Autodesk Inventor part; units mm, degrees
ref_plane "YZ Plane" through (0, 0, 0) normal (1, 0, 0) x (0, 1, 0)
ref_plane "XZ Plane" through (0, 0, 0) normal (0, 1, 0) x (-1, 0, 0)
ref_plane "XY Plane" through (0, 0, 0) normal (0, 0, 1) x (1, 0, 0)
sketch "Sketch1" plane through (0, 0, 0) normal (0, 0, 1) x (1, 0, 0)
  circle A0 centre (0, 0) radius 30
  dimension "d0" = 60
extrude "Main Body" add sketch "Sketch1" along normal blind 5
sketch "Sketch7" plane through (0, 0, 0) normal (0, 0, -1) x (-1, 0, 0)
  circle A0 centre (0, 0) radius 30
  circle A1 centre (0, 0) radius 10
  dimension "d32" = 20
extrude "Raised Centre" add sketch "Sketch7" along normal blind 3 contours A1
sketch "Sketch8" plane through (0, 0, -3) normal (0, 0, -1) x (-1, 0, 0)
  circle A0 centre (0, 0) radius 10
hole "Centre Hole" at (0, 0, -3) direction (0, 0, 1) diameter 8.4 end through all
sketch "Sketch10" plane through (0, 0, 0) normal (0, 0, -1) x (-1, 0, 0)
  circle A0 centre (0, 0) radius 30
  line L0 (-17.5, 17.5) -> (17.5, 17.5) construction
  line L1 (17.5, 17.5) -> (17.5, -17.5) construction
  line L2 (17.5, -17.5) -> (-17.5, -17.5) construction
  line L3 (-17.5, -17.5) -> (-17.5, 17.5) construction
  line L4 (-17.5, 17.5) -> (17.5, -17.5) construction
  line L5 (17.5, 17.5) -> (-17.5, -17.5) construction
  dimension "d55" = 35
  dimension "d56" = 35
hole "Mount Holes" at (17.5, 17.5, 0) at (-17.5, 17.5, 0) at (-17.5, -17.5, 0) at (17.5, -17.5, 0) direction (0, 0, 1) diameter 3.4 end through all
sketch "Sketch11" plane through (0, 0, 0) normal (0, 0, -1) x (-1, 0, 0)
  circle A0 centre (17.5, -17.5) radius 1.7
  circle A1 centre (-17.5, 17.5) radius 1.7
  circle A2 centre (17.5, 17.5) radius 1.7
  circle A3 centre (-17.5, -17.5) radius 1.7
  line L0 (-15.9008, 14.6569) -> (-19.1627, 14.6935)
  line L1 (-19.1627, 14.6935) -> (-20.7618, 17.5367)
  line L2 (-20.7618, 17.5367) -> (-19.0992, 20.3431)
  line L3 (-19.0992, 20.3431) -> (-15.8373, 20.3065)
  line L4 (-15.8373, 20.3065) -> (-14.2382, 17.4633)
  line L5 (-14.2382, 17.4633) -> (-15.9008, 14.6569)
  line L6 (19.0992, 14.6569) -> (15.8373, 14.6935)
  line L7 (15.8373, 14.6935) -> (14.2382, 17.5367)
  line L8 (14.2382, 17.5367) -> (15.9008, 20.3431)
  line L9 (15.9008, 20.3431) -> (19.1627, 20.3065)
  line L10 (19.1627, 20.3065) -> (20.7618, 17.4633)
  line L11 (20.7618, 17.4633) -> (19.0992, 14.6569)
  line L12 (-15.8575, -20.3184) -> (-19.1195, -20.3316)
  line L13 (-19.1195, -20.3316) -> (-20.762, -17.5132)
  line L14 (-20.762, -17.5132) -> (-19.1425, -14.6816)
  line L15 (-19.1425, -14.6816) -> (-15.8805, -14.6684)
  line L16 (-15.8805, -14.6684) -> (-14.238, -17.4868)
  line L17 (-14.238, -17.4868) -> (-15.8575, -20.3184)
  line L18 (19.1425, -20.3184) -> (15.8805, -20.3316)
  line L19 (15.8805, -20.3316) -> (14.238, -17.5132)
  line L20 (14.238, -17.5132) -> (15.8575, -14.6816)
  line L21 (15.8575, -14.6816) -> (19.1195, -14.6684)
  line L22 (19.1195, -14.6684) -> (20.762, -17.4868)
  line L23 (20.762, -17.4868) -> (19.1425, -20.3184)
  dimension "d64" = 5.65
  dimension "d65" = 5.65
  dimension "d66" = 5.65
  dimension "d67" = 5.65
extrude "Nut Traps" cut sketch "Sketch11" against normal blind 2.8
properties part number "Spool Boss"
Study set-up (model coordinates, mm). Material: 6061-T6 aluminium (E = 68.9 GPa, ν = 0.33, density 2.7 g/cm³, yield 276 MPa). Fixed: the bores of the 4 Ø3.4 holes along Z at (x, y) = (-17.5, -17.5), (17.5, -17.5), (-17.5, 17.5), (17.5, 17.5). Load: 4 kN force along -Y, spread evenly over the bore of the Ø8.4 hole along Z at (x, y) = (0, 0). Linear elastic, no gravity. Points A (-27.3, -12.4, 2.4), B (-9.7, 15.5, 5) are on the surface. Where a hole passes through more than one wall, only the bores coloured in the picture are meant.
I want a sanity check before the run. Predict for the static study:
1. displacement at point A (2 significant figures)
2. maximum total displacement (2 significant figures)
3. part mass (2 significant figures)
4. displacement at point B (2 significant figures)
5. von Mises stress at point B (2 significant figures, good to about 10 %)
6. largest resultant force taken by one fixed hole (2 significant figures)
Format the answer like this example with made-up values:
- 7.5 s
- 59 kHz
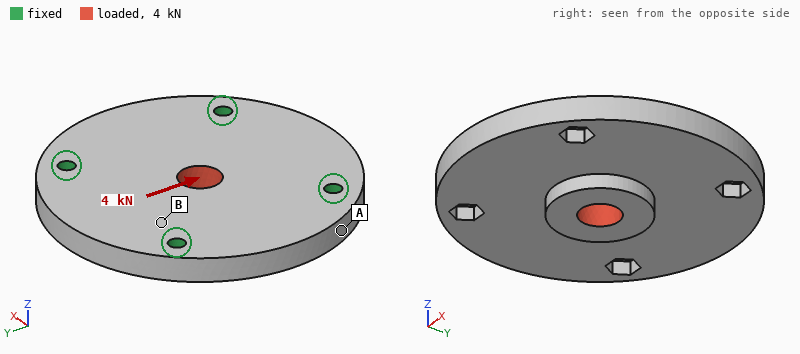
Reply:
- 2.3 µm
- 10 µm
- 38 g
- 4.5 µm
- 15 MPa
- 1.1 kN
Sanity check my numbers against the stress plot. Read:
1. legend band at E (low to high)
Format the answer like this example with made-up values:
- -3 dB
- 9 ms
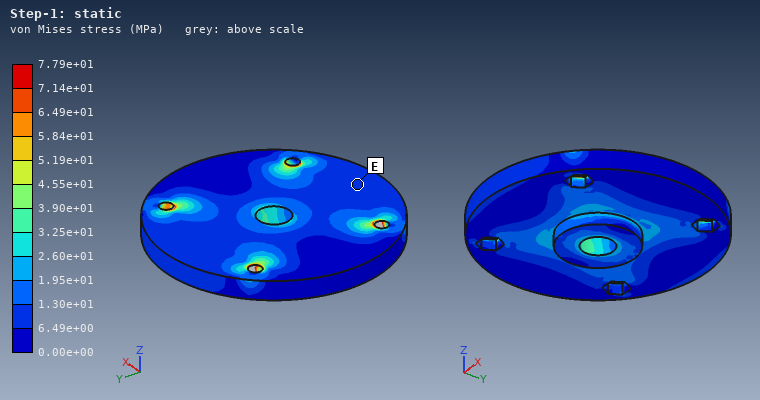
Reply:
- 6.49e+00 to 1.30e+01 MPa
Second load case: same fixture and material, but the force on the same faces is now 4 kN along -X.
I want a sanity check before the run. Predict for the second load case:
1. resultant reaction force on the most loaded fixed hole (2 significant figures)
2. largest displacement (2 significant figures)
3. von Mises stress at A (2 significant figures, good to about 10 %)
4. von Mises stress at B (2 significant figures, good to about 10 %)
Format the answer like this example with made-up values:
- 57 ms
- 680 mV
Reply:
- 1.1 kN
- 10 µm
- 9.4 MPa
- 17 MPa
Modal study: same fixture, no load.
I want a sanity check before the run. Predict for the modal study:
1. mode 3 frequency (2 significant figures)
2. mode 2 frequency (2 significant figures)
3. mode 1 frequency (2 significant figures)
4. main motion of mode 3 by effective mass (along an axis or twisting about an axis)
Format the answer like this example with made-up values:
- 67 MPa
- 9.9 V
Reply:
- 12 kHz
- 11 kHz
- 11 kHz
- twisting about Y
